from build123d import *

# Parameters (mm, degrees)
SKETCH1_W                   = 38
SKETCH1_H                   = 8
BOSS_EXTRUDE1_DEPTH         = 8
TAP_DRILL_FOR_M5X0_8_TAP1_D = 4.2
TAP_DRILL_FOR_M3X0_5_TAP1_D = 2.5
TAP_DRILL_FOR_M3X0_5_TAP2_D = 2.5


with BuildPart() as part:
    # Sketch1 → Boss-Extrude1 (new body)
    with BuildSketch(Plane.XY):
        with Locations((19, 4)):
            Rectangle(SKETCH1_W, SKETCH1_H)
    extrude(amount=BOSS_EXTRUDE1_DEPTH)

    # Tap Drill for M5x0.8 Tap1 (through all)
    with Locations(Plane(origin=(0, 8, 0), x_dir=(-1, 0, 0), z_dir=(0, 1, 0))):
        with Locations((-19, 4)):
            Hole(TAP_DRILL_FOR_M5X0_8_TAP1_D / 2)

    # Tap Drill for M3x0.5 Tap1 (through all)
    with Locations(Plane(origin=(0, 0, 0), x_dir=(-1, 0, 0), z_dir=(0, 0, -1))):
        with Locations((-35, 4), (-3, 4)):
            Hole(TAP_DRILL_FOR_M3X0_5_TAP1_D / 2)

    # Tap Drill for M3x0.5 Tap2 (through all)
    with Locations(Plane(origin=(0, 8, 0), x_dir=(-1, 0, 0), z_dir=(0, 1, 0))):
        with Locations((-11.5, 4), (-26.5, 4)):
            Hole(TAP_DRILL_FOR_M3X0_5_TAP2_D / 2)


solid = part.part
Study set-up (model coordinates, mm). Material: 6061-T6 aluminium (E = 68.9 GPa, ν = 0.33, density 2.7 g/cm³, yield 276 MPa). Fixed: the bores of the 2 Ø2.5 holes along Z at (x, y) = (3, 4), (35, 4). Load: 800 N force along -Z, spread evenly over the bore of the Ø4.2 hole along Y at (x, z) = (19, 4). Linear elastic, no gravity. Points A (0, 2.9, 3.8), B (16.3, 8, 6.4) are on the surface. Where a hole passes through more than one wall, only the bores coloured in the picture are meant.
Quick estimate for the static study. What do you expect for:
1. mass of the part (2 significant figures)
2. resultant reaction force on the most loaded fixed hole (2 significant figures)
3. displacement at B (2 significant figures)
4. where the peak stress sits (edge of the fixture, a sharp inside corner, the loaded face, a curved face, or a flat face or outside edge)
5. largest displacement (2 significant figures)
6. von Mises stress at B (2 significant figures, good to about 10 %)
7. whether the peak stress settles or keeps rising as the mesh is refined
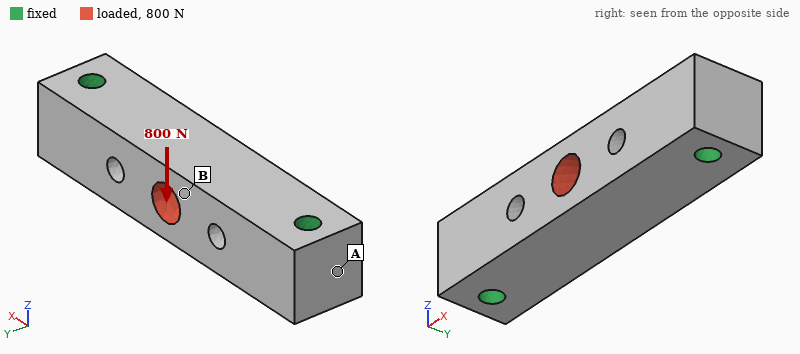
5.8 g
400 N
10 µm
edge of the fixture
11 µm
17 MPa
keeps rising
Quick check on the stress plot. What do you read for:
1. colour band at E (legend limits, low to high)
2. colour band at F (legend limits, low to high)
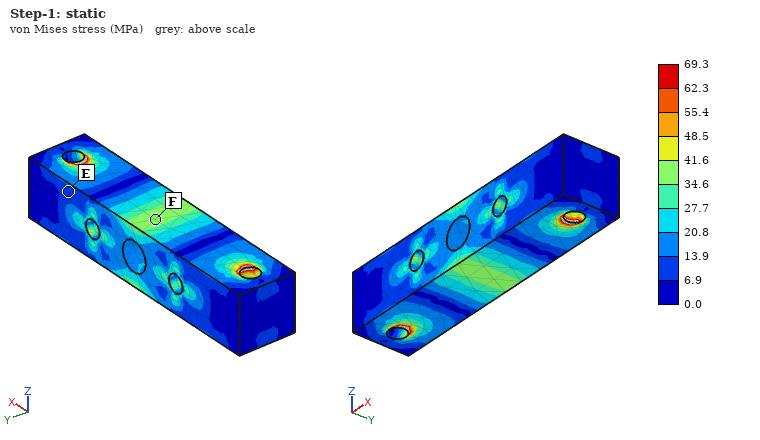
6.9 to 13.9 MPa
34.6 to 41.6 MPa
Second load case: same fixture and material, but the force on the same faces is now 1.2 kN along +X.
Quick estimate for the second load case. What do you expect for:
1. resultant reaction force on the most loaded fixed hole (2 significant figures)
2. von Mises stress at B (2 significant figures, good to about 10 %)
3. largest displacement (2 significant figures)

600 N
10 MPa
2.6 µm
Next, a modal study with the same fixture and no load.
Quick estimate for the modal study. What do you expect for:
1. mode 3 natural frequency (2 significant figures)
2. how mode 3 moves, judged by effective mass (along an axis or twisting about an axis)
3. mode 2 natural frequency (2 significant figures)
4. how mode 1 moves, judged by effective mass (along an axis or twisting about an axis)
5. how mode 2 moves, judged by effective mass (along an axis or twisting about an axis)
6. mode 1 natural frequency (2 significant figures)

45 kHz
twisting about X
31 kHz
along Y
along Z
25 kHz
